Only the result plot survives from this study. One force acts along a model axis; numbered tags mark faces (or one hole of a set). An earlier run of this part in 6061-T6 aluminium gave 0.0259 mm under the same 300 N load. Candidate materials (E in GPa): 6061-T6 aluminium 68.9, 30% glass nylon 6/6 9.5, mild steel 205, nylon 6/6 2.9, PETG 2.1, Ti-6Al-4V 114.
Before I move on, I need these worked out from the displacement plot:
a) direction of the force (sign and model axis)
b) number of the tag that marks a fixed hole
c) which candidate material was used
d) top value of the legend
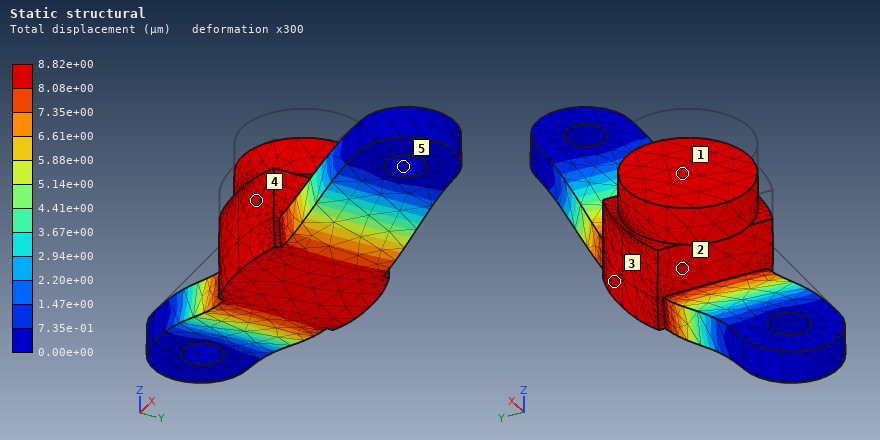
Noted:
-Z
5
mild steel
8.82e+00 µm
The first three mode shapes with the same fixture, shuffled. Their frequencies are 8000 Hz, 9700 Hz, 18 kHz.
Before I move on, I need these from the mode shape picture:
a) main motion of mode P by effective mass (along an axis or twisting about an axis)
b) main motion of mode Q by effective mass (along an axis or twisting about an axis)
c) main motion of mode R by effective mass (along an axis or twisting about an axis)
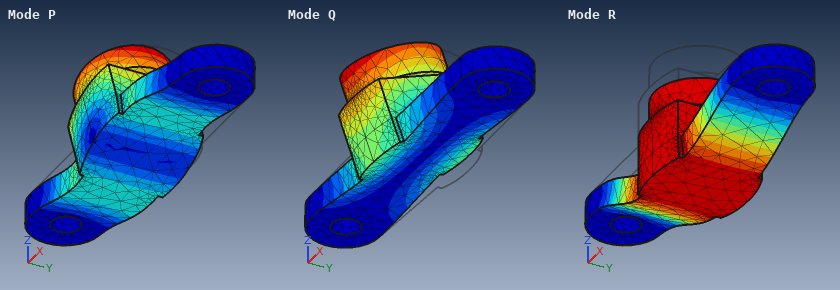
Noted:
along X
along Y
along Z
